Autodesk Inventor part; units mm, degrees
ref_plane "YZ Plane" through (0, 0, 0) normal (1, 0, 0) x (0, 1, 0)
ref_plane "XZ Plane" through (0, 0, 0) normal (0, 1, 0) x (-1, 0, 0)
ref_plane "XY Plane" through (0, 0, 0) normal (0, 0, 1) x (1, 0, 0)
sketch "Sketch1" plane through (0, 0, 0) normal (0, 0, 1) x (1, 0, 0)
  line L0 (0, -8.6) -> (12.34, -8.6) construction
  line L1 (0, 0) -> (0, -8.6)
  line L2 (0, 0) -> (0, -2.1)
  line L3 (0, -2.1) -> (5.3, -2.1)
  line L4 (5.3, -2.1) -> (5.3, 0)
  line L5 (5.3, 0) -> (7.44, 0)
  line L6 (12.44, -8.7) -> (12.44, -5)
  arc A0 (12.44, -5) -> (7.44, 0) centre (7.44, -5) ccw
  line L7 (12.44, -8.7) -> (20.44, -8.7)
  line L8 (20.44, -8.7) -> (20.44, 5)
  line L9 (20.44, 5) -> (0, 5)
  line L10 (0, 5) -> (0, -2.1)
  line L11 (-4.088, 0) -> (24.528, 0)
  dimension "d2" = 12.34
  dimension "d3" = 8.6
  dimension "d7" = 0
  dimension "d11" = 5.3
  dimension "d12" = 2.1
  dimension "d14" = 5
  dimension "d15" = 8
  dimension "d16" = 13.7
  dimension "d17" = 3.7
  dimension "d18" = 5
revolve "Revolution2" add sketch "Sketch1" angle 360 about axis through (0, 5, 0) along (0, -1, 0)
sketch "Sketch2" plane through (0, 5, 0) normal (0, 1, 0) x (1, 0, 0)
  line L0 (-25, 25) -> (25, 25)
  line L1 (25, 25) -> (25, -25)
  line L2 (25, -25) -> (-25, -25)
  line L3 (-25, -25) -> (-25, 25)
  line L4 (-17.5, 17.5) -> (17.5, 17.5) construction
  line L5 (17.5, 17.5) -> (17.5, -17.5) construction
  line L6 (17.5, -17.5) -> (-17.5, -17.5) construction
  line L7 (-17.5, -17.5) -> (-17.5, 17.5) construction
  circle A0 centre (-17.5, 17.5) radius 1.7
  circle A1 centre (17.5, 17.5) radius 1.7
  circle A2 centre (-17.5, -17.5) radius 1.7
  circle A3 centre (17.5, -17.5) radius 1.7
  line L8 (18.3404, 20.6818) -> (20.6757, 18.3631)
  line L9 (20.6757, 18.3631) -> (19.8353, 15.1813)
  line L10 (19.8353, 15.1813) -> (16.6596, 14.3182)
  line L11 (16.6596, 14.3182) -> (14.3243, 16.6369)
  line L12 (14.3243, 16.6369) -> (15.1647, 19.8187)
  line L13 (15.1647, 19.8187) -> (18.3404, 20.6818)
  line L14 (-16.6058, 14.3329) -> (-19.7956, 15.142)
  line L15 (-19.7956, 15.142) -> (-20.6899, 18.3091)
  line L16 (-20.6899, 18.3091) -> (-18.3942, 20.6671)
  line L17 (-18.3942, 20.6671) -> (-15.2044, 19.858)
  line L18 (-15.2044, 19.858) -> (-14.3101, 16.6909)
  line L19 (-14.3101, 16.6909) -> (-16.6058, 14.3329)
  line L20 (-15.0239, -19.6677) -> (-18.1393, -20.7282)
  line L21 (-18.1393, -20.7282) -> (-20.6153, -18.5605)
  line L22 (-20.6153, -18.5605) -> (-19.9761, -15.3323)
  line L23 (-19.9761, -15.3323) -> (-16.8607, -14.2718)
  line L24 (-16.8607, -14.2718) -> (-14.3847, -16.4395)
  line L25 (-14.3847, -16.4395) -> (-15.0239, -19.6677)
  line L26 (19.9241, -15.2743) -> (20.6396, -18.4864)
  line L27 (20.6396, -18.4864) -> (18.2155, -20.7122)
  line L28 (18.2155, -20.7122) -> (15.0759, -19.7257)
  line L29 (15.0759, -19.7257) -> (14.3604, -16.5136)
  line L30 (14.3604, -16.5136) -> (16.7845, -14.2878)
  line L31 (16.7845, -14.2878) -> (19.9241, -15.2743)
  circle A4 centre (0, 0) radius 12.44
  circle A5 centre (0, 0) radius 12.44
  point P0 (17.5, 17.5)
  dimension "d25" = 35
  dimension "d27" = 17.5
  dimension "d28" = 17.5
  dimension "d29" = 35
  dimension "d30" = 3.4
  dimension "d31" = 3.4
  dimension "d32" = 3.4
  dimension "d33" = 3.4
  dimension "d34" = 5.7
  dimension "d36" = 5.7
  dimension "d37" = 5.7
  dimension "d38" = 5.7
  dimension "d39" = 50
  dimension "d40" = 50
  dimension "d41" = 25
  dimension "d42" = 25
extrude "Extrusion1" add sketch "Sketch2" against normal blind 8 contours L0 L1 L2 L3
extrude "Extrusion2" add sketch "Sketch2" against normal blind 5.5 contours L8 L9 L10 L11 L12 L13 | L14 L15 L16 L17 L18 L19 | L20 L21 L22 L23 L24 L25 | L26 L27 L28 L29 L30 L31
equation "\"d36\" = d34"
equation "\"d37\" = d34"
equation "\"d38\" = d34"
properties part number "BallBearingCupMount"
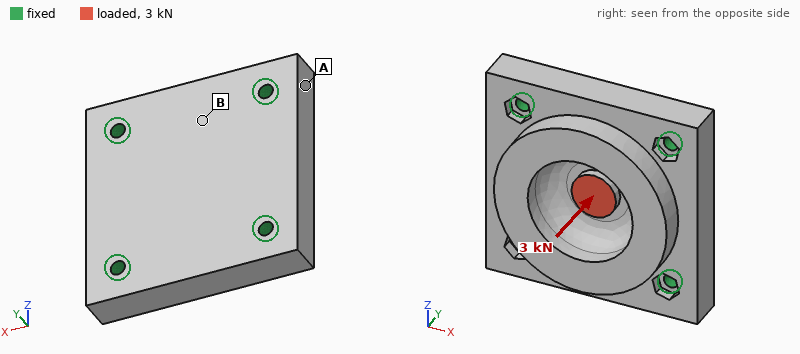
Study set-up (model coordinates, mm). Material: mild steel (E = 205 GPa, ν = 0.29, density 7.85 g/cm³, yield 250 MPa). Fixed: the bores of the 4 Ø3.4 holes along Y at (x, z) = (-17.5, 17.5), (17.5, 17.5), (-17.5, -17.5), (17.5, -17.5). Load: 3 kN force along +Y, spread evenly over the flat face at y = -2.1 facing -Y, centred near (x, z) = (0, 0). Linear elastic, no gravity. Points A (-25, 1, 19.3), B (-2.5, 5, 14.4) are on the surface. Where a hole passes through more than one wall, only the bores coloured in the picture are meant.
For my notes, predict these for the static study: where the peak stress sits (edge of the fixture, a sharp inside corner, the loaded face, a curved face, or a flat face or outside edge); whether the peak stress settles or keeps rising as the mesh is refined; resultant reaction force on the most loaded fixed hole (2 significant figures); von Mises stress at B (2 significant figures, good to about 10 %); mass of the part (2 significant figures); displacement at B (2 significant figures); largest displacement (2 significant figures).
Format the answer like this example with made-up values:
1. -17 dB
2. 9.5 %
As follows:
1. edge of the fixture
2. keeps rising
3. 860 N
4. 15 MPa
5. 180 g
6. 2.5 µm
7. 7.2 µm
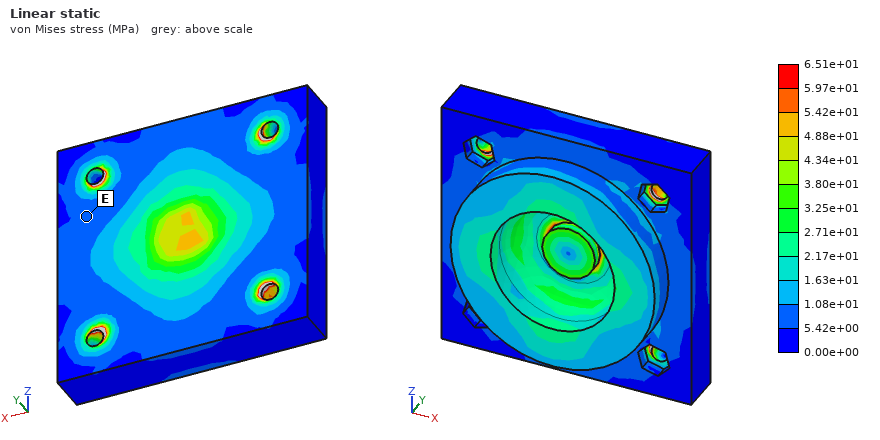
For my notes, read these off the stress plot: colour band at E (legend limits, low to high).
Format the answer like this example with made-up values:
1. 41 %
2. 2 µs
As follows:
1. 5.42e+00 to 1.08e+01 MPa
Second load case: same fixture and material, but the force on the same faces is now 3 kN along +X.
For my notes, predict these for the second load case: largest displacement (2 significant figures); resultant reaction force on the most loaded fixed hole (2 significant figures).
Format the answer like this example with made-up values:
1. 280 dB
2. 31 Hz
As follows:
1. 5.5 µm
2. 850 N
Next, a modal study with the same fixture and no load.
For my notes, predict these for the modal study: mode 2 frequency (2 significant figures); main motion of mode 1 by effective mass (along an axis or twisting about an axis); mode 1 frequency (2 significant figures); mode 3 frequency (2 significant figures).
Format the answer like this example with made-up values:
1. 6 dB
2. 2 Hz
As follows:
1. 23 kHz
2. along Y
3. 18 kHz
4. 24 kHz
